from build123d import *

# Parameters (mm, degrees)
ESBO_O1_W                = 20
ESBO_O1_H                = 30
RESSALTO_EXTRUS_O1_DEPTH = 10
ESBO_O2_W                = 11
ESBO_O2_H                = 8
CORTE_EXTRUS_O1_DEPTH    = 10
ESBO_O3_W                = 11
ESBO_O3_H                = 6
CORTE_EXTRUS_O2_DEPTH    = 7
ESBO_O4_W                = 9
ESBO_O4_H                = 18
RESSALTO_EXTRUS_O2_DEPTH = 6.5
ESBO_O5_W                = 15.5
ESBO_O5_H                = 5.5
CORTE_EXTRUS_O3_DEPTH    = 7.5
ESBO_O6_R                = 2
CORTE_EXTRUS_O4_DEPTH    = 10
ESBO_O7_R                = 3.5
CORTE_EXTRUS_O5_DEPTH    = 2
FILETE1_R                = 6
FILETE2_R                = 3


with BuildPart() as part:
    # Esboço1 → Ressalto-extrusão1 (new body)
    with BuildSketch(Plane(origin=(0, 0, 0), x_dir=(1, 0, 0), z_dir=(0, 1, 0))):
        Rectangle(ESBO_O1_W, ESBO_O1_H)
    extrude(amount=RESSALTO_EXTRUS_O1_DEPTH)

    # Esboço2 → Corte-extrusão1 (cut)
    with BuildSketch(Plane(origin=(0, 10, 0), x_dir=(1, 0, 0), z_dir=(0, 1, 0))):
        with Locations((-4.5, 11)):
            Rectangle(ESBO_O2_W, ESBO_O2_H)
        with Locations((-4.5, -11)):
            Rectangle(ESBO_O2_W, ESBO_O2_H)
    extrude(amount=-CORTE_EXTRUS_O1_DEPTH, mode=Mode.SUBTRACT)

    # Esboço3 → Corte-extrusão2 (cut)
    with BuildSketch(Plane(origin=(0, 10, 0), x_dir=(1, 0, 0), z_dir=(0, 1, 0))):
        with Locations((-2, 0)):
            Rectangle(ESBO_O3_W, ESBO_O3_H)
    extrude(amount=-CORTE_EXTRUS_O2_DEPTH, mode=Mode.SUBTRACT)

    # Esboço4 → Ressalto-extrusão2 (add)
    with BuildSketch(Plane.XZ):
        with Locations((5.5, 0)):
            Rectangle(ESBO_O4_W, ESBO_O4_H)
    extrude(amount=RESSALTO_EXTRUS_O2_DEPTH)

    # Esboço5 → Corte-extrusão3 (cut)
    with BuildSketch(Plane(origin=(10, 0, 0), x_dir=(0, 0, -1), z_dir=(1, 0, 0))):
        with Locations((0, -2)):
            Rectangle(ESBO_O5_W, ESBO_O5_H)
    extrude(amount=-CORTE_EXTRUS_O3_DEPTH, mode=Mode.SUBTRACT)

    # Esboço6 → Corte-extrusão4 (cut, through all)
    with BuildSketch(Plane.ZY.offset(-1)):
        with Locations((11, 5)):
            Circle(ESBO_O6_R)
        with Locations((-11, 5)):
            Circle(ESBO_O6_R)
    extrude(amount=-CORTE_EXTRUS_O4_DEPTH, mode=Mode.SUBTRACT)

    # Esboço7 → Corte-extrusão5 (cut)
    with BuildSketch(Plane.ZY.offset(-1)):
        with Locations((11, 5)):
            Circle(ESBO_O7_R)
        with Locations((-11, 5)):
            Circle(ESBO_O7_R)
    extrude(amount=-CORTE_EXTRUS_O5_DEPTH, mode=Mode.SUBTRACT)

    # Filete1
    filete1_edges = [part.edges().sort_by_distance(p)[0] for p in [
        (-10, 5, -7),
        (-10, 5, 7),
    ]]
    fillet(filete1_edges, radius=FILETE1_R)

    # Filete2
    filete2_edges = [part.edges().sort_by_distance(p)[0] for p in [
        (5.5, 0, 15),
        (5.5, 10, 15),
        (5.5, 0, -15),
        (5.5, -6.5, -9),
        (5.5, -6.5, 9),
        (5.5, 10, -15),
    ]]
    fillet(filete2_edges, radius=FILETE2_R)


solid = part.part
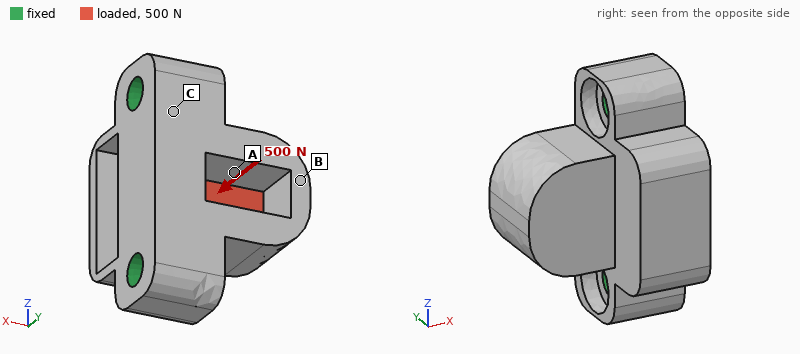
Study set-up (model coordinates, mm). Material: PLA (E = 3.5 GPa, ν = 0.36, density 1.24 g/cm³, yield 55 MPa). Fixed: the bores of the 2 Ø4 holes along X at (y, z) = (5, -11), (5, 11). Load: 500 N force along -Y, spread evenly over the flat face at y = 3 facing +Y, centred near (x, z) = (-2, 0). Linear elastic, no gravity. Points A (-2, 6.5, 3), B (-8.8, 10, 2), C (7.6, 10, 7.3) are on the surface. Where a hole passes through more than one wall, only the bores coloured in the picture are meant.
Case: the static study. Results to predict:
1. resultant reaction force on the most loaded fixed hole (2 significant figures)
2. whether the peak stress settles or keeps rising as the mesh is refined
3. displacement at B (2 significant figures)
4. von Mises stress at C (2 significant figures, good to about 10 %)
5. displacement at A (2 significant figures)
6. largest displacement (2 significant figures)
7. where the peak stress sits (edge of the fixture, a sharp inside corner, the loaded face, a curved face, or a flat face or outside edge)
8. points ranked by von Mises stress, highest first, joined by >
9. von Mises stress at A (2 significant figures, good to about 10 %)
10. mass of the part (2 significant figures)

250 N
keeps rising
0.22 mm
13 MPa
0.11 mm
0.23 mm
edge of the fixture
C > A > B
7.2 MPa
4.5 g
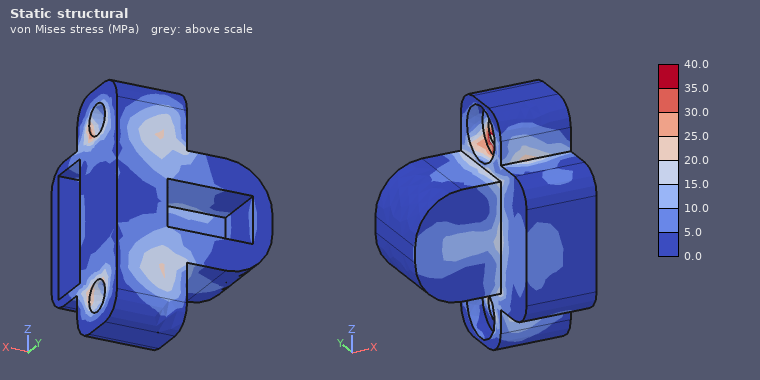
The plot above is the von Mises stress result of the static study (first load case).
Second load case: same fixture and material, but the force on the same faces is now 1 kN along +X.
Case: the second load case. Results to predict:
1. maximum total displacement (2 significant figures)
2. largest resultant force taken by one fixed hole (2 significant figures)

0.13 mm
520 N
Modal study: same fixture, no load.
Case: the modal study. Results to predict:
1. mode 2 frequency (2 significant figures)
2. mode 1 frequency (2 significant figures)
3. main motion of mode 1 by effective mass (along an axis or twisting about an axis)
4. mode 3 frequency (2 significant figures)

9000 Hz
6000 Hz
along Y
9300 Hz
